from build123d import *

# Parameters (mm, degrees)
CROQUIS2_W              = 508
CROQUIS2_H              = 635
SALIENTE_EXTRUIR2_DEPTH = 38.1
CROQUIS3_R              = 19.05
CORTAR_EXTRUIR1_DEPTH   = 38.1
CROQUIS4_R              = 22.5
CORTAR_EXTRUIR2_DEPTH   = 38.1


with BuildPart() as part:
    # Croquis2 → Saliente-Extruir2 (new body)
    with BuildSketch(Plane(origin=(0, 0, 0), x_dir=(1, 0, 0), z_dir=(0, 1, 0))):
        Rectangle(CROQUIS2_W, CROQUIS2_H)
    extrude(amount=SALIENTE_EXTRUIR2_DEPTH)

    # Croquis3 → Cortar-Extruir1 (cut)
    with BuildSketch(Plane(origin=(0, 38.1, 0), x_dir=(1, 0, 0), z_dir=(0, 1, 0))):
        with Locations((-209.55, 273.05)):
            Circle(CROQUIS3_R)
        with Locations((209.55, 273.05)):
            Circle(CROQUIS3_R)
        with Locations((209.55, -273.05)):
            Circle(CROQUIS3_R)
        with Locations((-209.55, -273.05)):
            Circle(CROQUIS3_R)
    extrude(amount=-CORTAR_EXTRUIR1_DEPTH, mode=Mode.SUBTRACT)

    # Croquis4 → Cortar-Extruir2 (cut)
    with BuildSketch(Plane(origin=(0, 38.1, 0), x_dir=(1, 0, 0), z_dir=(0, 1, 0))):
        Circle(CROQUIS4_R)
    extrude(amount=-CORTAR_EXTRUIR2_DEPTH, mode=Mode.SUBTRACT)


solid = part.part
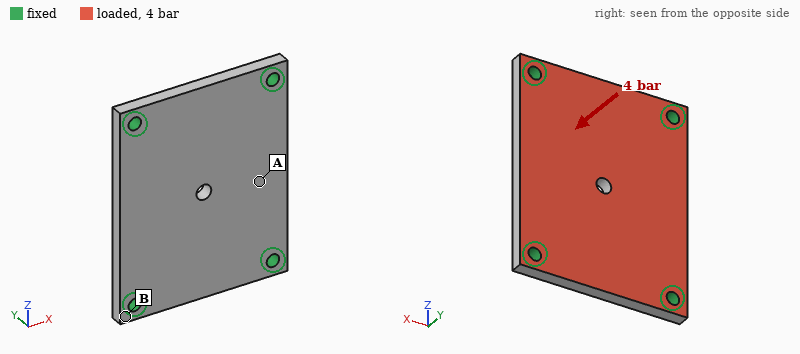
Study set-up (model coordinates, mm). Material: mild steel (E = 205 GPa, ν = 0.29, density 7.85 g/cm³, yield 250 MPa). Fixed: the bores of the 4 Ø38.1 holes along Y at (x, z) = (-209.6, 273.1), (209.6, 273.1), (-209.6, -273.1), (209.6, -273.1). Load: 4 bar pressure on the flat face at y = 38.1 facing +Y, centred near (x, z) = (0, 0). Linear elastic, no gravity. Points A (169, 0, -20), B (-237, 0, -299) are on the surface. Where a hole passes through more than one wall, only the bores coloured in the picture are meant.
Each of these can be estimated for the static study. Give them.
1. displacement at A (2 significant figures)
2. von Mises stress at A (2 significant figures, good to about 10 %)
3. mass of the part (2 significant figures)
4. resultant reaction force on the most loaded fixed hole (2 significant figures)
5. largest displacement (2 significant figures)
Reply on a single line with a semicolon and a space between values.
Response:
0.14 mm; 23 MPa; 95 kg; 32 kN; 0.18 mm
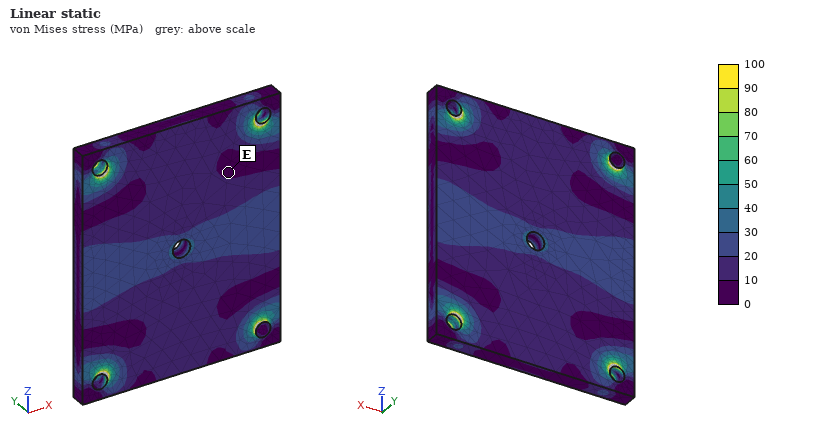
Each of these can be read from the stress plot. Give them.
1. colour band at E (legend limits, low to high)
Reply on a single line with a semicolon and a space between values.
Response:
0 to 10 MPa
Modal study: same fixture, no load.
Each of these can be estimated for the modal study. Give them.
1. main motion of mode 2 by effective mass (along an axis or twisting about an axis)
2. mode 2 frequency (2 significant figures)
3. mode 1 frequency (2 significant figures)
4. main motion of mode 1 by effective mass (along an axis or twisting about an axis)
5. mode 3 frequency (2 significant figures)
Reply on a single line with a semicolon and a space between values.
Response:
twisting about Z; 810 Hz; 530 Hz; along Y; 1100 Hz
